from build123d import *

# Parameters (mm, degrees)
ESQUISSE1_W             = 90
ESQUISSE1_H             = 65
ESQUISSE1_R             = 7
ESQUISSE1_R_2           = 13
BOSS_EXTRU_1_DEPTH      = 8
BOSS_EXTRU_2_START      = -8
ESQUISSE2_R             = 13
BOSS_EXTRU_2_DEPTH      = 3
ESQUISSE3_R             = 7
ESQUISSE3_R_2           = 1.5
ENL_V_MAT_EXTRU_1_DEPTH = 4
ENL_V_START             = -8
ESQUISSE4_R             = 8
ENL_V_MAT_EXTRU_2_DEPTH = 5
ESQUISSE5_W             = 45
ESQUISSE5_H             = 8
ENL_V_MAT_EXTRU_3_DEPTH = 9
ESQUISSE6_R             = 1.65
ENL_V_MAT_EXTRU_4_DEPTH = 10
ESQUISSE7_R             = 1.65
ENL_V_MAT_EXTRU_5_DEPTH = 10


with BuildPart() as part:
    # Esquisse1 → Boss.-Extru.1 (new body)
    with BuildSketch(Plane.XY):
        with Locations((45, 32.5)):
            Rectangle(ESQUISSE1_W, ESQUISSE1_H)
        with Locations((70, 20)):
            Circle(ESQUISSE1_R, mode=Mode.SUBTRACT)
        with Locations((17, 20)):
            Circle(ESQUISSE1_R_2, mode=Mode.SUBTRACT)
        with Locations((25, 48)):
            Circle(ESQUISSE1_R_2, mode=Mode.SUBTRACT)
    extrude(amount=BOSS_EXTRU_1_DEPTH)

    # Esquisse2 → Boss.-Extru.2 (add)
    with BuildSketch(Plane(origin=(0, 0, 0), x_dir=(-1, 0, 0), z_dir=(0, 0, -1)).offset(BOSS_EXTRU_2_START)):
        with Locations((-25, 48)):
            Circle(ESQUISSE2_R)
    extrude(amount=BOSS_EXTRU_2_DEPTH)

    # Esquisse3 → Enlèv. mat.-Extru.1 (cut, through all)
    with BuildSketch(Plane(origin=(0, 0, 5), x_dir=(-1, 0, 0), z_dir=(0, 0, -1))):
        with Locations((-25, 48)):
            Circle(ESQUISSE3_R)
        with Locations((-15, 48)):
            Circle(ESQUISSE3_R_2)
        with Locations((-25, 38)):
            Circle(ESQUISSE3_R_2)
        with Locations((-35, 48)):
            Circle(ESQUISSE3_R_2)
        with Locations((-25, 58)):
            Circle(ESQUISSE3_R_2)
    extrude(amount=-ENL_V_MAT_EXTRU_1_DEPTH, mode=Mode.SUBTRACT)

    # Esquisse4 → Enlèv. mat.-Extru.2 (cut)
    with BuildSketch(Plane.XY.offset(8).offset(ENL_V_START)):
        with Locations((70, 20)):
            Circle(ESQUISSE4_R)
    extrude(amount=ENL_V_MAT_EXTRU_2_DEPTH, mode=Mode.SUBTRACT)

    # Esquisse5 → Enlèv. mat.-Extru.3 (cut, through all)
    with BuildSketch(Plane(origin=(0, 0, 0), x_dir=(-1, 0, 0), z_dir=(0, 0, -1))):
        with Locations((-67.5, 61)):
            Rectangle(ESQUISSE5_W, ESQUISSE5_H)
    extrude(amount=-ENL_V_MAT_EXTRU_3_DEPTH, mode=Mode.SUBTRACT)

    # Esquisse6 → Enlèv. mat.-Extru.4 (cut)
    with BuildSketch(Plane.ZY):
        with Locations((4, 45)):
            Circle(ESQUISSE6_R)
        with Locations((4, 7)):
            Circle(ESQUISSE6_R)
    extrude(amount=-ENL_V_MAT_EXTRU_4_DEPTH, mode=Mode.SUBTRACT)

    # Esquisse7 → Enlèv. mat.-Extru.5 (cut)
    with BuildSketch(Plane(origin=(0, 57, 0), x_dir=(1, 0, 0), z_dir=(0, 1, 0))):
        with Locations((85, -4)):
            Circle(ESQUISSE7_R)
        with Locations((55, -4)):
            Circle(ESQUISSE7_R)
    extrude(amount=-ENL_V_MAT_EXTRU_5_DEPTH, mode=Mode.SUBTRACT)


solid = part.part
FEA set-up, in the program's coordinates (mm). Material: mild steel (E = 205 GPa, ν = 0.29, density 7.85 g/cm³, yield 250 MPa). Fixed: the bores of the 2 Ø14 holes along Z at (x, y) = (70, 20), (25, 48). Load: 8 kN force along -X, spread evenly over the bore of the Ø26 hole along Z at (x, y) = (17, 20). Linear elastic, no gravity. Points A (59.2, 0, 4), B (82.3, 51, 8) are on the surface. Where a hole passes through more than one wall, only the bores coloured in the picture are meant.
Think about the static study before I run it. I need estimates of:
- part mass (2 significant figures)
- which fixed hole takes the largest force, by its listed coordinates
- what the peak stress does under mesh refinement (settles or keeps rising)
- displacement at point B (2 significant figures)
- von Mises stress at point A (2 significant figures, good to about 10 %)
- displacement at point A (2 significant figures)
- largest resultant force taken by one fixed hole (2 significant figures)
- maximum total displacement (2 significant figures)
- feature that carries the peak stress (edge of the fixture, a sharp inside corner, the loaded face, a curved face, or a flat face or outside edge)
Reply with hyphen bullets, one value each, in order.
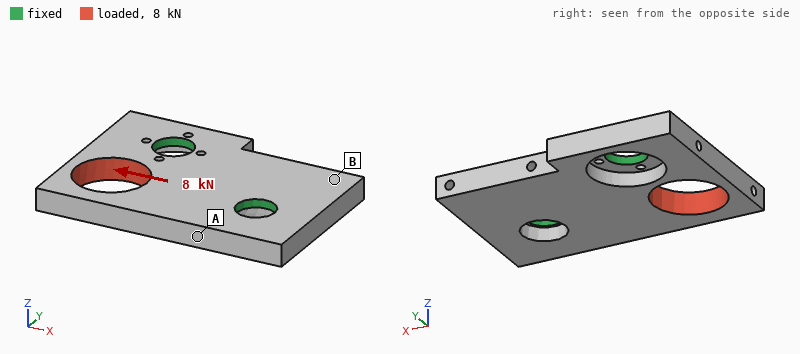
- 270 g
- (70, 20)
- keeps rising
- 4.8 µm
- 22 MPa
- 6.1 µm
- 5.3 kN
- 30 µm
- edge of the fixture
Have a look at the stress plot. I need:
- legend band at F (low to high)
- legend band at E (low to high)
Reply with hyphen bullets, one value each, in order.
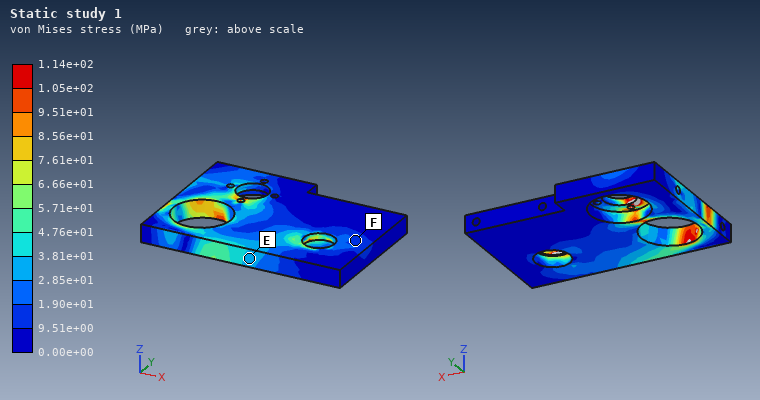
- 9.51e+00 to 1.90e+01 MPa
- 2.85e+01 to 3.81e+01 MPa
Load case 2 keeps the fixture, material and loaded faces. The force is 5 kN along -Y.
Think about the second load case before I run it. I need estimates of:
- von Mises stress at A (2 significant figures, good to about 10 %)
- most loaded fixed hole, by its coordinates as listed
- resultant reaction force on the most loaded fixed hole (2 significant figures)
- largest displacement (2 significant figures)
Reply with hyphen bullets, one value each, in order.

- 10 MPa
- (25, 48)
- 4.7 kN
- 25 µm
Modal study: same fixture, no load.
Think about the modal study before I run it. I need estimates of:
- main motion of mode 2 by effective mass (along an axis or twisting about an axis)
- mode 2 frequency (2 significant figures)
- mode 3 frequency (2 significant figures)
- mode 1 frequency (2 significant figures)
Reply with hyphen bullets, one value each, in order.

- along Z
- 5200 Hz
- 6400 Hz
- 3000 Hz
